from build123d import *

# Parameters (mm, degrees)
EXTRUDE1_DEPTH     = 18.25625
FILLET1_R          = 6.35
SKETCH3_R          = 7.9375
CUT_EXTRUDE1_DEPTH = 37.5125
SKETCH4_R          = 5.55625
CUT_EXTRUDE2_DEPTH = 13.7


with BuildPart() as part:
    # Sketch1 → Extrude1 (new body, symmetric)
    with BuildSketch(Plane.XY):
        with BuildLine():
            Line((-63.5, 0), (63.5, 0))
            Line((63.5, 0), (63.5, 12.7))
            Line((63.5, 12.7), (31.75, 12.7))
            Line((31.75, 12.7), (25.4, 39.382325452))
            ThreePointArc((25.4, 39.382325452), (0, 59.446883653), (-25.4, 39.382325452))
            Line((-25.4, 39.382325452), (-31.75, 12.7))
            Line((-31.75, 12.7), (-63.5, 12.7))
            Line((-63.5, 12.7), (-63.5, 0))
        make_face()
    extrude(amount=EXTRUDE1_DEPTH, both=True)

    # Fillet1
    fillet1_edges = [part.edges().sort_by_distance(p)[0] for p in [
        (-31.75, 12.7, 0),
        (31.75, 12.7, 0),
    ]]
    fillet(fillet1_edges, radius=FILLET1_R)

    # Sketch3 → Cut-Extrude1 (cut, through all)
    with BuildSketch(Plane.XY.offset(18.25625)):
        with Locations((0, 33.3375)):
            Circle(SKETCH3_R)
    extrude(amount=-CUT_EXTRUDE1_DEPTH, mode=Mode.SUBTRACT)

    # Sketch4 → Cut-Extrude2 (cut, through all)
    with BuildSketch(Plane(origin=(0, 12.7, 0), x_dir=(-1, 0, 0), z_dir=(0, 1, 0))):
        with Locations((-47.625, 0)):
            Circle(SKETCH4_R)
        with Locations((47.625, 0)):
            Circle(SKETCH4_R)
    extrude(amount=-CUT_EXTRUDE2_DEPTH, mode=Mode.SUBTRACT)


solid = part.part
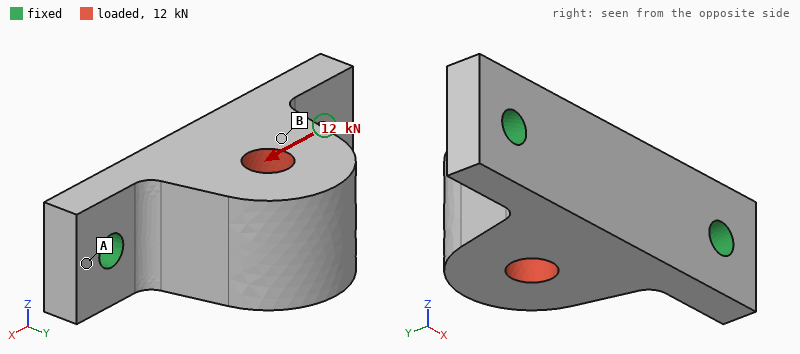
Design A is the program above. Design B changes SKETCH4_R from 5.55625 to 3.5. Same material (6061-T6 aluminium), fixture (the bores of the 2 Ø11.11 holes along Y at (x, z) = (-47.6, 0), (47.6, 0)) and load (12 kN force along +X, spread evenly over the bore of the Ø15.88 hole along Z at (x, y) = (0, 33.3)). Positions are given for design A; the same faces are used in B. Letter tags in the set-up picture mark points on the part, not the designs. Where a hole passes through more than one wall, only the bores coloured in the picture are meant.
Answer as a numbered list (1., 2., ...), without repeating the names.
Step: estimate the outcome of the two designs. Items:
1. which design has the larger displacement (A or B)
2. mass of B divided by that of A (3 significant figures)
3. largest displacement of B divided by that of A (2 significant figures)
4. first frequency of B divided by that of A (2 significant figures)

1. B
2. 1.01
3. 1.2
4. 0.87
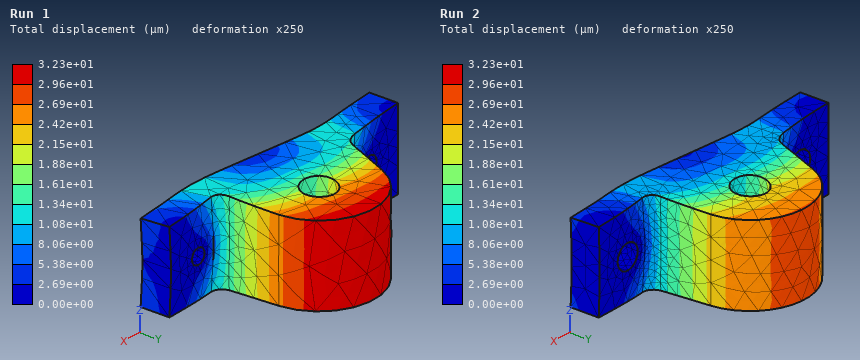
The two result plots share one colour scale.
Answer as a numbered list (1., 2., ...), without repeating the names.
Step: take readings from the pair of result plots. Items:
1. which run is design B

1. Run 1
